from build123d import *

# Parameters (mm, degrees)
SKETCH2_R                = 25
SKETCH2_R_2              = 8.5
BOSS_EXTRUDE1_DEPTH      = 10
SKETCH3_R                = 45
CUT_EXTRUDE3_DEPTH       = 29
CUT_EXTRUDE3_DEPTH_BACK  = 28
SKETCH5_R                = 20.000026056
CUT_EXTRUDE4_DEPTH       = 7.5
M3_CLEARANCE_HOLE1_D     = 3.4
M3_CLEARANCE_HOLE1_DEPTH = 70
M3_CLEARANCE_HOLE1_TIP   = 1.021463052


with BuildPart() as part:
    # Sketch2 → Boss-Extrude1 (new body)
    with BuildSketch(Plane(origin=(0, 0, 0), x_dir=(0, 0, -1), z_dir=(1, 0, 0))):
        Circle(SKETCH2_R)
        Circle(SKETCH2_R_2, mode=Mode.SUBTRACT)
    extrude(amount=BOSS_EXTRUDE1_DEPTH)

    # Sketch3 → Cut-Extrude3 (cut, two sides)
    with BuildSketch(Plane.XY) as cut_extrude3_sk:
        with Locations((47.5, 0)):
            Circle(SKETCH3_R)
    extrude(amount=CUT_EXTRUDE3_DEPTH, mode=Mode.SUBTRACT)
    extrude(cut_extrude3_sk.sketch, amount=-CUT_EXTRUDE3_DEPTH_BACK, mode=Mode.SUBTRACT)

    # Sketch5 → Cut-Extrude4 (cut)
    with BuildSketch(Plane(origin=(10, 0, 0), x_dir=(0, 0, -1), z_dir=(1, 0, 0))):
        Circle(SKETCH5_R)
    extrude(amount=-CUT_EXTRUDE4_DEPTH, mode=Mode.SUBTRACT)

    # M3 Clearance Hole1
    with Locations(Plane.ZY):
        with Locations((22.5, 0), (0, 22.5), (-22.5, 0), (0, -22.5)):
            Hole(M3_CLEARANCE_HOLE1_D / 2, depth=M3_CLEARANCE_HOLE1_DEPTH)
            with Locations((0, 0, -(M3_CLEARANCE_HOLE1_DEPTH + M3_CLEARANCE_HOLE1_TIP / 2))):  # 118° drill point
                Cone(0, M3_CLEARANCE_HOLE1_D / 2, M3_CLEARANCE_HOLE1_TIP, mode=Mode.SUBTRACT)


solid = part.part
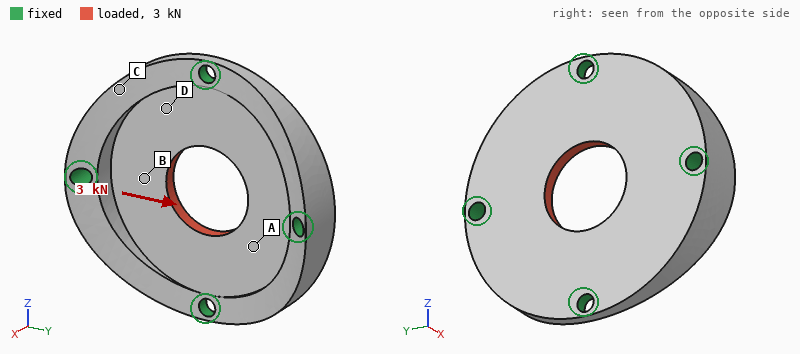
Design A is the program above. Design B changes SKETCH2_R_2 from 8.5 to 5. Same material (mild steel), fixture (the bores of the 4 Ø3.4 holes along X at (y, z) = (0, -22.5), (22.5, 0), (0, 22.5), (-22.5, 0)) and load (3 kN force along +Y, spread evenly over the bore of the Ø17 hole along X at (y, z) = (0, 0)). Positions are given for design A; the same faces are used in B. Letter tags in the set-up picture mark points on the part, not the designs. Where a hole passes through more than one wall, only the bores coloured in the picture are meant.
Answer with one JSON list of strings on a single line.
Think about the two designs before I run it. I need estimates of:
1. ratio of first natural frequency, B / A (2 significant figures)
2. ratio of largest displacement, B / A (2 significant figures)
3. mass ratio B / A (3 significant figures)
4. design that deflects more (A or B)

["0.84", "1.2", "1.06", "B"]
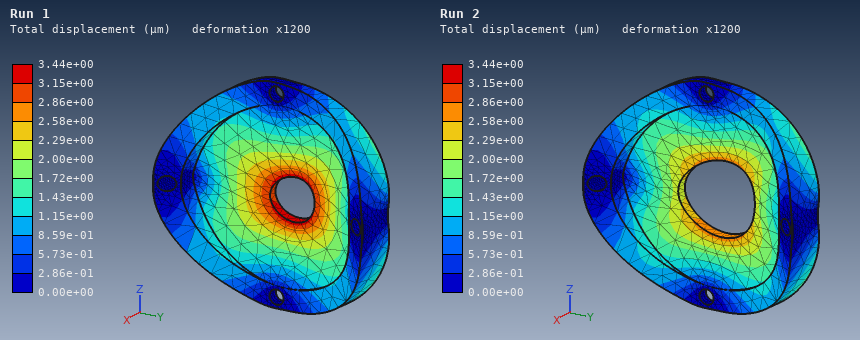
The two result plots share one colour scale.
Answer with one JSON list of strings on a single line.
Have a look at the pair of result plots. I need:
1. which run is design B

["Run 1"]
